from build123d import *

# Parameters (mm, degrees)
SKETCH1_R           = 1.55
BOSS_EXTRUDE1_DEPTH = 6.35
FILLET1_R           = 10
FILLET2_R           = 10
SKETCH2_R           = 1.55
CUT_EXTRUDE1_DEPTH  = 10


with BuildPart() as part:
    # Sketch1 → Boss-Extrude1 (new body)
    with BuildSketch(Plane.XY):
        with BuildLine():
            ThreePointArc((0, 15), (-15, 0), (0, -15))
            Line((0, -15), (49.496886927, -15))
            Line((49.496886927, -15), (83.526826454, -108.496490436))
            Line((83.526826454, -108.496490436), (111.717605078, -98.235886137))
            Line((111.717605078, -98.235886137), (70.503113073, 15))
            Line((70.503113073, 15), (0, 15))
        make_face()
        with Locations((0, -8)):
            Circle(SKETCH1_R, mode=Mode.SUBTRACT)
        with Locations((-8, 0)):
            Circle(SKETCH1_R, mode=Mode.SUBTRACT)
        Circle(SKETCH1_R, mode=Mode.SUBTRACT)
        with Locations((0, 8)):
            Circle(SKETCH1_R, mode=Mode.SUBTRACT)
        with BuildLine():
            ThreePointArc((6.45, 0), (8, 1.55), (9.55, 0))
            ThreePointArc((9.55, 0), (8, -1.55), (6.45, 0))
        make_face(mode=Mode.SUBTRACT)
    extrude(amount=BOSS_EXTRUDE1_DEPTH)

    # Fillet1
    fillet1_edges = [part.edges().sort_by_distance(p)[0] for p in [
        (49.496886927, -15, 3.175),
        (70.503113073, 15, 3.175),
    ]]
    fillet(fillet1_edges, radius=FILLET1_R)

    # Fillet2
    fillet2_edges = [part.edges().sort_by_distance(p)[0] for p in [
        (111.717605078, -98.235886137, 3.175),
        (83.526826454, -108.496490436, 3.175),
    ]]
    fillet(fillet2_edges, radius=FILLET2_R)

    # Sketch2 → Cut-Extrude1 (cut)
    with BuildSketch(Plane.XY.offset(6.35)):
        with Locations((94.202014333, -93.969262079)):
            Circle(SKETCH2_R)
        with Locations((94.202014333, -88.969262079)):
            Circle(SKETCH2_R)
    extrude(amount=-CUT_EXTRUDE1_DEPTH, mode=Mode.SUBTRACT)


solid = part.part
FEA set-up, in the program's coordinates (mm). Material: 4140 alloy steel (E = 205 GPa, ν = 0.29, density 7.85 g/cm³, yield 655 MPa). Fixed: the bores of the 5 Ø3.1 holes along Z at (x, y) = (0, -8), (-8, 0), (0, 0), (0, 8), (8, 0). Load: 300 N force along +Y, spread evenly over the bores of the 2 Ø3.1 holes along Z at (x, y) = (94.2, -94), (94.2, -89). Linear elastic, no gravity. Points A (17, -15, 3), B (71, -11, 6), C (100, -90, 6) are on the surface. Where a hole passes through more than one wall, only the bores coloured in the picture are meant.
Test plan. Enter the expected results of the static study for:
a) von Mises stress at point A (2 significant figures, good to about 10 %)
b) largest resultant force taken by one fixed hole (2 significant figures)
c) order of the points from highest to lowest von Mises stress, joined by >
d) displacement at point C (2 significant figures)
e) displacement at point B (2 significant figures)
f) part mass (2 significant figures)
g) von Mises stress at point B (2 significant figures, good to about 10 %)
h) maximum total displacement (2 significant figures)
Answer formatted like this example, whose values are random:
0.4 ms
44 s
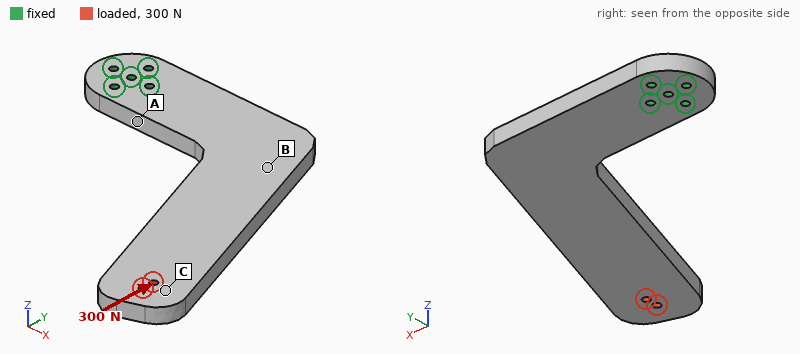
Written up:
25 MPa
1.1 kN
A > B > C
59 µm
21 µm
270 g
5.7 MPa
65 µm
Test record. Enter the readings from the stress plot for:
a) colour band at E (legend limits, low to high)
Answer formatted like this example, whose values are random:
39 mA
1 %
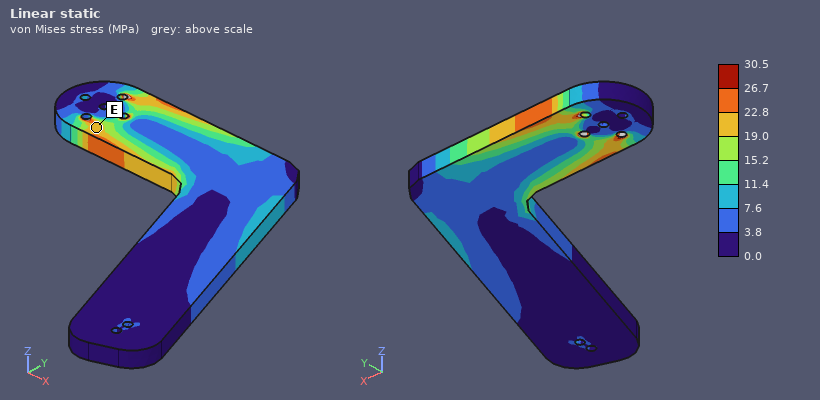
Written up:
19.0 to 22.8 MPa
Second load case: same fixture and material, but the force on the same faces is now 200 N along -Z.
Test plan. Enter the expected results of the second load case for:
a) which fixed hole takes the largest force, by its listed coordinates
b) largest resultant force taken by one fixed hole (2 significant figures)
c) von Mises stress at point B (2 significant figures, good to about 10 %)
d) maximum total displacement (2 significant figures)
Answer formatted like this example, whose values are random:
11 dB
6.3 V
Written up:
(8, 0)
1.1 kN
72 MPa
1.4 mm
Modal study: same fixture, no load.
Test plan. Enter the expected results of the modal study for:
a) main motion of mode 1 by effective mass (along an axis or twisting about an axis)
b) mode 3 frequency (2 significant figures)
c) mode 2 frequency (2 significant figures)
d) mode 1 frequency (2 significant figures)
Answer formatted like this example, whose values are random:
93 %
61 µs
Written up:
along Z
1000 Hz
970 Hz
250 Hz
